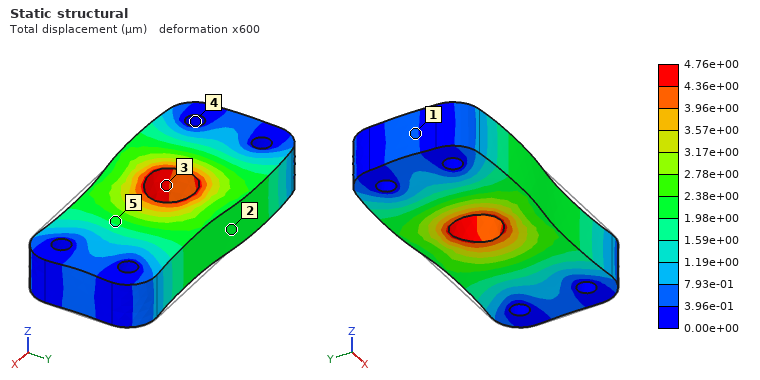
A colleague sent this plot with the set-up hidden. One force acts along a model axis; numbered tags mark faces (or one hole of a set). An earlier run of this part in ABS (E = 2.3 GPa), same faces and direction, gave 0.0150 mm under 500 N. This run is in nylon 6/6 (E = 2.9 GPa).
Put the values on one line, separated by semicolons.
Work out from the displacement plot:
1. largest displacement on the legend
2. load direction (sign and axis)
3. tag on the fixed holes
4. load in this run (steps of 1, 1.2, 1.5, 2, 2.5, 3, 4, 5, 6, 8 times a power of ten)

4.76e+00 µm; -X; 4; 200 N
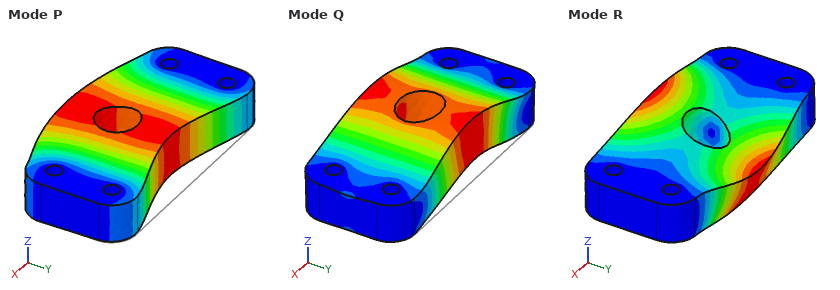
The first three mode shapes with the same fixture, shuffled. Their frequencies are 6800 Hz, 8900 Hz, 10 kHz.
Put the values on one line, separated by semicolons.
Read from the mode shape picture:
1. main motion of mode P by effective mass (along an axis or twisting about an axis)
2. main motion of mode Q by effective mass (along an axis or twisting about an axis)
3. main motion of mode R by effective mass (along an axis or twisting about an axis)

along Y; along Z; twisting about X
